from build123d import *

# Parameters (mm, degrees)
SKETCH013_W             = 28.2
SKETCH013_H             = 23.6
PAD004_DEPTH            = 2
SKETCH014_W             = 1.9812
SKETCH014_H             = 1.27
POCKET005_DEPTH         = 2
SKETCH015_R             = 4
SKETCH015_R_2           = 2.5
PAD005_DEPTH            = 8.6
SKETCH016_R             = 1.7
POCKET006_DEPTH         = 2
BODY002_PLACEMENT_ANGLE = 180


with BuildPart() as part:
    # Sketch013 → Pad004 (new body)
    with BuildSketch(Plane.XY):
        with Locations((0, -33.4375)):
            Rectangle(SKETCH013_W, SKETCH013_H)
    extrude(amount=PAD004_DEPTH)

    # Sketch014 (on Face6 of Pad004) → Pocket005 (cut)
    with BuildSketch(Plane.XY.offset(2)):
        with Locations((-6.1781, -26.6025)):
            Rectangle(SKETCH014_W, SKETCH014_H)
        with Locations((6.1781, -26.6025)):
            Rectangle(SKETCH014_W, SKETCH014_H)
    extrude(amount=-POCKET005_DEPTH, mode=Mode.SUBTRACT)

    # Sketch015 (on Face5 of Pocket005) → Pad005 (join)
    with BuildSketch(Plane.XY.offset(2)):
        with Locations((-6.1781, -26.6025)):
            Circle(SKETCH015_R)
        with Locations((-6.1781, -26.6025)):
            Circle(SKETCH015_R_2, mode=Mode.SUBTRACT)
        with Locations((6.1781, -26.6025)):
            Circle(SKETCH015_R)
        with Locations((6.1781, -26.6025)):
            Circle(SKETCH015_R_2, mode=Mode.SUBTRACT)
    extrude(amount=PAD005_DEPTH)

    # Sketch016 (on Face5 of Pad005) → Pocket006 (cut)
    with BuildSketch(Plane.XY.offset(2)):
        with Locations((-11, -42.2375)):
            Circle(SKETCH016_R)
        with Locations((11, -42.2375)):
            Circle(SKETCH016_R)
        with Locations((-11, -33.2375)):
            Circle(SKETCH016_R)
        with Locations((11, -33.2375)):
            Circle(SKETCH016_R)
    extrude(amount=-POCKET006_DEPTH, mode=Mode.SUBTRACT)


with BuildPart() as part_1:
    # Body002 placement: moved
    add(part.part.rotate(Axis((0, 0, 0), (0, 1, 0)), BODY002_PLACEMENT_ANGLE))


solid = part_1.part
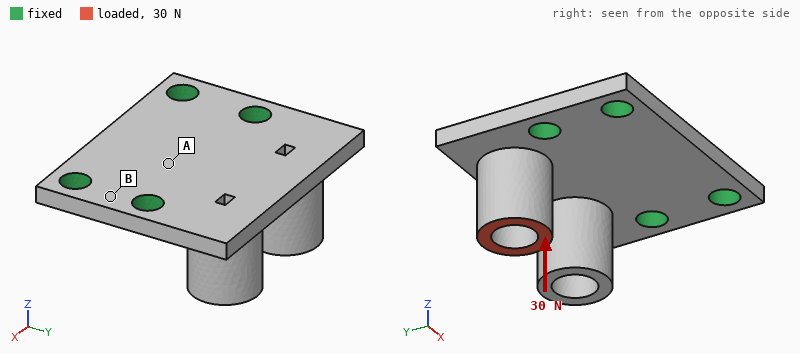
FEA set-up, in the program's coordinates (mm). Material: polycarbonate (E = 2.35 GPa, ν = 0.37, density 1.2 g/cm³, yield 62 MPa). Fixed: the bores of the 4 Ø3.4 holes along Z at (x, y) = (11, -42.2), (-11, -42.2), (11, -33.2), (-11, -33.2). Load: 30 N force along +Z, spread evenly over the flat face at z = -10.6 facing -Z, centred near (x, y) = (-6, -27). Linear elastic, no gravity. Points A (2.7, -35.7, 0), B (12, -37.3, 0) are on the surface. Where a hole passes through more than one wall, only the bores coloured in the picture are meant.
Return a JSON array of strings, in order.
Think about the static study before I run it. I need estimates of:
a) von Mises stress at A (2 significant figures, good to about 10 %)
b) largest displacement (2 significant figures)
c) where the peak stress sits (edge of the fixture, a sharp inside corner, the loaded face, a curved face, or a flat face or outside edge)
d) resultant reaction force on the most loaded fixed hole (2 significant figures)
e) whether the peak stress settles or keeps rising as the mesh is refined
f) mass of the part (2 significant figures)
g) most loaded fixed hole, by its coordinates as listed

["2.8 MPa", "0.25 mm", "edge of the fixture", "27 N", "keeps rising", "2.1 g", "(-11, -33.2)"]
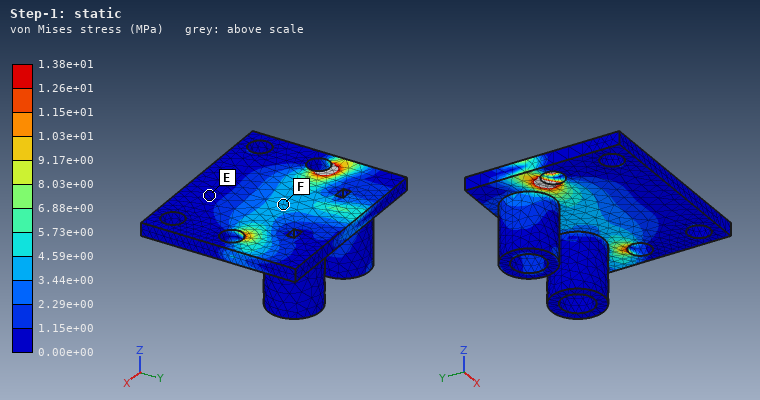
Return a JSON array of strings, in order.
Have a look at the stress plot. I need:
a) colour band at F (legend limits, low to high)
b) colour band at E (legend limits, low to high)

["3.44e+00 to 4.59e+00 MPa", "0.00e+00 to 1.15e+00 MPa"]
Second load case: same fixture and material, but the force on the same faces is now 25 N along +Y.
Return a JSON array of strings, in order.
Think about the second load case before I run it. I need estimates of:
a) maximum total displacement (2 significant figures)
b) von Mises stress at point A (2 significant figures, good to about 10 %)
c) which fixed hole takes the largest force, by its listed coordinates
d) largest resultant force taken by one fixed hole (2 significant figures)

["0.44 mm", "3.5 MPa", "(-11, -33.2)", "16 N"]
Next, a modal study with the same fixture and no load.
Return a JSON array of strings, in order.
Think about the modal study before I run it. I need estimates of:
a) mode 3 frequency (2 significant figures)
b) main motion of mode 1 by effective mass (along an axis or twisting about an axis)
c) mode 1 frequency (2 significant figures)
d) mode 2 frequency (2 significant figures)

["4200 Hz", "along Z", "2000 Hz", "3700 Hz"]
